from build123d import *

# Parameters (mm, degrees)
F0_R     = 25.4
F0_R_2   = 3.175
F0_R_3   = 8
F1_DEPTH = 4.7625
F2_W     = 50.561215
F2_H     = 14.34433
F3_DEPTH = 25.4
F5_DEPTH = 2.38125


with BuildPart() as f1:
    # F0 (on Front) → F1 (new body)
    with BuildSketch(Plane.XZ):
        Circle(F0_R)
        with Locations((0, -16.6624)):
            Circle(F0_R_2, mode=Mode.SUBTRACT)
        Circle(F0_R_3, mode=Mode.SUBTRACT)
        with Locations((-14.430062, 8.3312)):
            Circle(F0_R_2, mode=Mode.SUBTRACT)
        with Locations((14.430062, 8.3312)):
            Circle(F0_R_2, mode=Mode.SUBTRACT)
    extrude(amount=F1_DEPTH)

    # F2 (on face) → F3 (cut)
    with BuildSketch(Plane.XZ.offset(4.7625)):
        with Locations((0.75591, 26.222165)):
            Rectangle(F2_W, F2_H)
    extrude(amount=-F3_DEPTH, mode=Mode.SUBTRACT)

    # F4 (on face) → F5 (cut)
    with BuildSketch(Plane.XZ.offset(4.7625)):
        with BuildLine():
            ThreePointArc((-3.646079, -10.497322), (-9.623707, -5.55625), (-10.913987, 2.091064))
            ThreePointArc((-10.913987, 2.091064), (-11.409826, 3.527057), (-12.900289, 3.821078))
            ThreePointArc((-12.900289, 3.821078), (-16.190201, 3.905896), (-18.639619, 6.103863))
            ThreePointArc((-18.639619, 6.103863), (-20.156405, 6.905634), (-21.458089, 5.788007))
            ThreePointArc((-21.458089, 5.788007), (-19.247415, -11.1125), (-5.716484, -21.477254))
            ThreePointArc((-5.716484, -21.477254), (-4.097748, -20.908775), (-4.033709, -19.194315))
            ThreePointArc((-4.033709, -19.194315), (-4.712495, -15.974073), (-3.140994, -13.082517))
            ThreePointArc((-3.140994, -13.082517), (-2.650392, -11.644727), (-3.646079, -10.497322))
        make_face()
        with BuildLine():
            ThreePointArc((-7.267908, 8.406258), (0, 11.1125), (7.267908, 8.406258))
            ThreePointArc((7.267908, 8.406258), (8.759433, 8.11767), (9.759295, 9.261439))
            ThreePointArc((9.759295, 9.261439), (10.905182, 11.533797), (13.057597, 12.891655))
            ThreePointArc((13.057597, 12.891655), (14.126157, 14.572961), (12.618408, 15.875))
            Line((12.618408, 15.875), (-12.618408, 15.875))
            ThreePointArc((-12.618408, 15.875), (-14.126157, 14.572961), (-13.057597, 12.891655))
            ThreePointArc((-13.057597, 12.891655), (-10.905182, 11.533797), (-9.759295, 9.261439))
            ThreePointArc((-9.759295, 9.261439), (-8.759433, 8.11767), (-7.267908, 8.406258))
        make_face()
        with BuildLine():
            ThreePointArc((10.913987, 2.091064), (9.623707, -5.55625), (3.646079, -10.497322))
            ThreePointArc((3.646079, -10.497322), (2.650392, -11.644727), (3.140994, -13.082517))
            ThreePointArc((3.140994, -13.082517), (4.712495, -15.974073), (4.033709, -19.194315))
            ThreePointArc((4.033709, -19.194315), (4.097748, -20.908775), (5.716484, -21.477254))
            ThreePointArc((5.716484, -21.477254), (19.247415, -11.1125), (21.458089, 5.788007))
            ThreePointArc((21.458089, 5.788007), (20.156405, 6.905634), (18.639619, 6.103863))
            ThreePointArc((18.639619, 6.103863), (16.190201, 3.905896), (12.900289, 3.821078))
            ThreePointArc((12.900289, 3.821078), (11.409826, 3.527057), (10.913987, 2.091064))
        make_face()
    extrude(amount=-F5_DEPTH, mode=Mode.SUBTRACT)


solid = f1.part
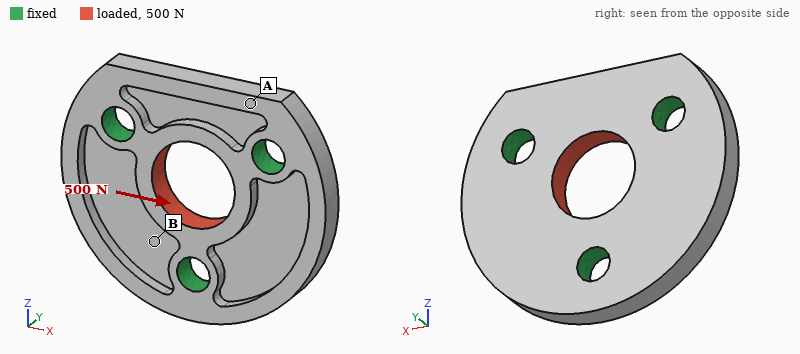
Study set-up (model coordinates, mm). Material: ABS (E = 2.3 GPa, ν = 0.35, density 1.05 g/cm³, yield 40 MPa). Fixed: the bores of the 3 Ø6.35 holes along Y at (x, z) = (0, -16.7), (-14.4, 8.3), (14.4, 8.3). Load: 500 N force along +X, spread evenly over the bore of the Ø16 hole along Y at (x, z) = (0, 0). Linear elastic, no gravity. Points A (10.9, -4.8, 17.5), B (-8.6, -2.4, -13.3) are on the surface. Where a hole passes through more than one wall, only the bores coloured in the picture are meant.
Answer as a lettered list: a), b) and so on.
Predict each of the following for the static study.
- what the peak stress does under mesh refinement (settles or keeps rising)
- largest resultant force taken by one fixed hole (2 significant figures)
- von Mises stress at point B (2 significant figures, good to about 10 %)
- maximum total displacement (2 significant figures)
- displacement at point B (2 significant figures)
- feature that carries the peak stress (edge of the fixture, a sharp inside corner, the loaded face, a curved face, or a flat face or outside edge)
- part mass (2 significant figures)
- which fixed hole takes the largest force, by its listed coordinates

a) keeps rising
b) 180 N
c) 2.7 MPa
d) 42 µm
e) 14 µm
f) edge of the fixture
g) 6.1 g
h) (0, -16.7)
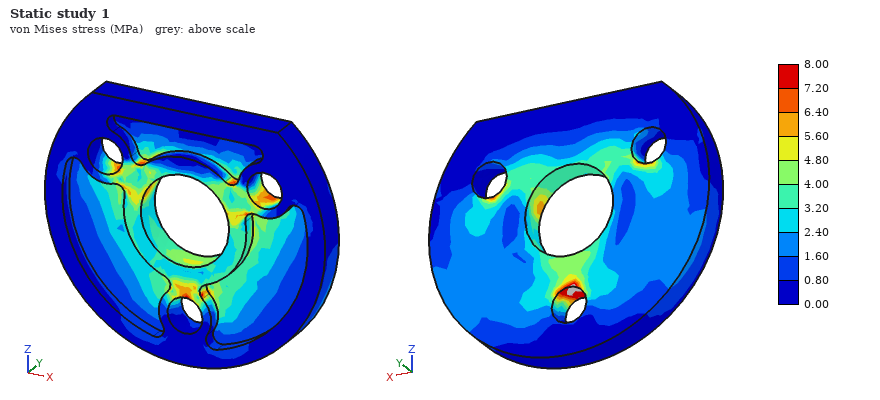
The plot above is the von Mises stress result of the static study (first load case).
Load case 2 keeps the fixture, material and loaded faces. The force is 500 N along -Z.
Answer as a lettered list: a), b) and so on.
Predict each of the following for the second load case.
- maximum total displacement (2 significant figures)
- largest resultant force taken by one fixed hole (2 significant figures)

a) 52 µm
b) 170 N
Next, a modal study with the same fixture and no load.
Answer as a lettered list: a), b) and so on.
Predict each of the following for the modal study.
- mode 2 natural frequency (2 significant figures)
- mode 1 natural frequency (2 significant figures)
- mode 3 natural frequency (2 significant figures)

a) 3300 Hz
b) 3200 Hz
c) 6100 Hz
